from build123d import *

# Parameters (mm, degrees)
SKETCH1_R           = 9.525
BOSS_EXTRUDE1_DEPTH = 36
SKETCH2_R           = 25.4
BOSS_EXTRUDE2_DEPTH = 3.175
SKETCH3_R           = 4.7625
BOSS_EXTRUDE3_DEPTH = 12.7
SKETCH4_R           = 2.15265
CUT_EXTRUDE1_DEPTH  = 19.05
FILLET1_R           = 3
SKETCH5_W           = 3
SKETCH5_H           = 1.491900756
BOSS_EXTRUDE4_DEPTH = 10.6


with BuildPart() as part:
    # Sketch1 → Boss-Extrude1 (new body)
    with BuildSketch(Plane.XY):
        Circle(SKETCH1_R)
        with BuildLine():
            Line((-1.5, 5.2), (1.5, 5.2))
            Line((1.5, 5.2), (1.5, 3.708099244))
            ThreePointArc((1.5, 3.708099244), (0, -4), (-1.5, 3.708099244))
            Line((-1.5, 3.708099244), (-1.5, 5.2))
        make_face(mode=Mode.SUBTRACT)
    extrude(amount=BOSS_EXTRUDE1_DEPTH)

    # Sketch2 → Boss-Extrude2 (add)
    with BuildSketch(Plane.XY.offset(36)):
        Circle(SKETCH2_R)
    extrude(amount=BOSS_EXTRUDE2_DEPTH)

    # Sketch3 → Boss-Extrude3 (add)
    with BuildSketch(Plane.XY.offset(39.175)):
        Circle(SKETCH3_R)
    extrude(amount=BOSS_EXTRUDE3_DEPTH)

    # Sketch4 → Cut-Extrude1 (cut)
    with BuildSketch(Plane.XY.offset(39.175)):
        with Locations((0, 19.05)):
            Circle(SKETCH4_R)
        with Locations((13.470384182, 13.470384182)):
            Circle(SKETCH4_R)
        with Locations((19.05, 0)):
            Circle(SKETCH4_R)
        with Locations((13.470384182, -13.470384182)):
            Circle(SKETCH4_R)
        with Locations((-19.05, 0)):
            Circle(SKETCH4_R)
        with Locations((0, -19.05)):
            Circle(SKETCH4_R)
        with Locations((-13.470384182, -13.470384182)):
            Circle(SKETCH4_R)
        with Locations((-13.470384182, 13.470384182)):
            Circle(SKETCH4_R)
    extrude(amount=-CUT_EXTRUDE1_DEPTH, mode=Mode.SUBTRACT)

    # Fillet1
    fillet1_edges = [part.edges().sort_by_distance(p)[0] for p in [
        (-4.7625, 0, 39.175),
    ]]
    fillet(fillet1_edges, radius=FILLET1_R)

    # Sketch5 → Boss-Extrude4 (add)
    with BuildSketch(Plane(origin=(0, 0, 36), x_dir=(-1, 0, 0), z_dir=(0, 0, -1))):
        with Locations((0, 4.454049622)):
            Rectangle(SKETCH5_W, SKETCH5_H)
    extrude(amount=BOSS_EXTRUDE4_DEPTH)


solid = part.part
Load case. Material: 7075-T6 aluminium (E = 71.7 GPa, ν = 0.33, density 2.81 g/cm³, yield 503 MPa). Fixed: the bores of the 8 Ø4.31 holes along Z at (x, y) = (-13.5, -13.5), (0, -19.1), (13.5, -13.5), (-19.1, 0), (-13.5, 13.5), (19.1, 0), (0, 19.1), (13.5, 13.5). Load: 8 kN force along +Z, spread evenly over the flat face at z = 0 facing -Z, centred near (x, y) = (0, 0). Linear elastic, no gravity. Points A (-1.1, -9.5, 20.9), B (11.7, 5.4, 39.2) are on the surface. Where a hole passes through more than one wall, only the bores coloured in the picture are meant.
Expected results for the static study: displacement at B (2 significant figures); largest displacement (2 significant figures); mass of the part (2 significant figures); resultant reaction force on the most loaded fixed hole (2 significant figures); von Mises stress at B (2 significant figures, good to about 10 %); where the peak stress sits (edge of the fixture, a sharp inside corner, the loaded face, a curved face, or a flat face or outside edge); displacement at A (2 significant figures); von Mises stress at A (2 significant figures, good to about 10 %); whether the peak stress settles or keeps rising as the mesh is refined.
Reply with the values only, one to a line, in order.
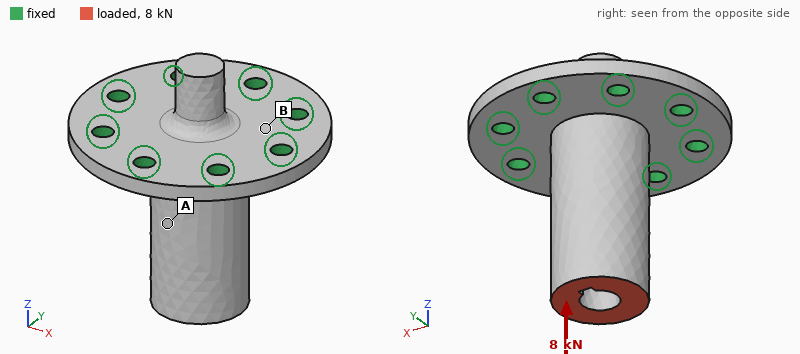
29 µm
70 µm
43 g
1.1 kN
72 MPa
edge of the fixture
60 µm
33 MPa
keeps rising
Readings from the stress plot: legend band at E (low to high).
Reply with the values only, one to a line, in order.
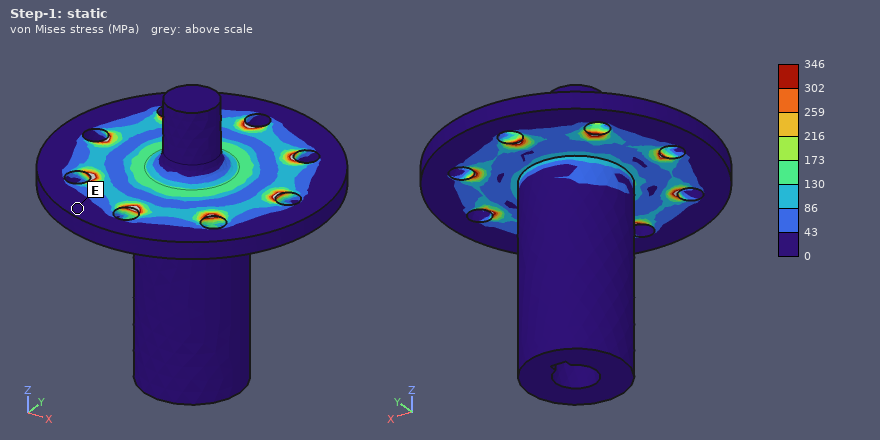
0 to 43 MPa
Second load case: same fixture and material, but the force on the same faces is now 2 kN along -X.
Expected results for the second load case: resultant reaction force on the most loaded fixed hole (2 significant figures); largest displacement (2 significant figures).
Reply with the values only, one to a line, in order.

1.4 kN
0.29 mm
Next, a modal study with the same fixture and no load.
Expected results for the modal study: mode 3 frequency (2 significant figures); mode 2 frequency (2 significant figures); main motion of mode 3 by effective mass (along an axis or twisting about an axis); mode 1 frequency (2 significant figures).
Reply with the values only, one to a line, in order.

11 kHz
4800 Hz
along Z
4800 Hz
